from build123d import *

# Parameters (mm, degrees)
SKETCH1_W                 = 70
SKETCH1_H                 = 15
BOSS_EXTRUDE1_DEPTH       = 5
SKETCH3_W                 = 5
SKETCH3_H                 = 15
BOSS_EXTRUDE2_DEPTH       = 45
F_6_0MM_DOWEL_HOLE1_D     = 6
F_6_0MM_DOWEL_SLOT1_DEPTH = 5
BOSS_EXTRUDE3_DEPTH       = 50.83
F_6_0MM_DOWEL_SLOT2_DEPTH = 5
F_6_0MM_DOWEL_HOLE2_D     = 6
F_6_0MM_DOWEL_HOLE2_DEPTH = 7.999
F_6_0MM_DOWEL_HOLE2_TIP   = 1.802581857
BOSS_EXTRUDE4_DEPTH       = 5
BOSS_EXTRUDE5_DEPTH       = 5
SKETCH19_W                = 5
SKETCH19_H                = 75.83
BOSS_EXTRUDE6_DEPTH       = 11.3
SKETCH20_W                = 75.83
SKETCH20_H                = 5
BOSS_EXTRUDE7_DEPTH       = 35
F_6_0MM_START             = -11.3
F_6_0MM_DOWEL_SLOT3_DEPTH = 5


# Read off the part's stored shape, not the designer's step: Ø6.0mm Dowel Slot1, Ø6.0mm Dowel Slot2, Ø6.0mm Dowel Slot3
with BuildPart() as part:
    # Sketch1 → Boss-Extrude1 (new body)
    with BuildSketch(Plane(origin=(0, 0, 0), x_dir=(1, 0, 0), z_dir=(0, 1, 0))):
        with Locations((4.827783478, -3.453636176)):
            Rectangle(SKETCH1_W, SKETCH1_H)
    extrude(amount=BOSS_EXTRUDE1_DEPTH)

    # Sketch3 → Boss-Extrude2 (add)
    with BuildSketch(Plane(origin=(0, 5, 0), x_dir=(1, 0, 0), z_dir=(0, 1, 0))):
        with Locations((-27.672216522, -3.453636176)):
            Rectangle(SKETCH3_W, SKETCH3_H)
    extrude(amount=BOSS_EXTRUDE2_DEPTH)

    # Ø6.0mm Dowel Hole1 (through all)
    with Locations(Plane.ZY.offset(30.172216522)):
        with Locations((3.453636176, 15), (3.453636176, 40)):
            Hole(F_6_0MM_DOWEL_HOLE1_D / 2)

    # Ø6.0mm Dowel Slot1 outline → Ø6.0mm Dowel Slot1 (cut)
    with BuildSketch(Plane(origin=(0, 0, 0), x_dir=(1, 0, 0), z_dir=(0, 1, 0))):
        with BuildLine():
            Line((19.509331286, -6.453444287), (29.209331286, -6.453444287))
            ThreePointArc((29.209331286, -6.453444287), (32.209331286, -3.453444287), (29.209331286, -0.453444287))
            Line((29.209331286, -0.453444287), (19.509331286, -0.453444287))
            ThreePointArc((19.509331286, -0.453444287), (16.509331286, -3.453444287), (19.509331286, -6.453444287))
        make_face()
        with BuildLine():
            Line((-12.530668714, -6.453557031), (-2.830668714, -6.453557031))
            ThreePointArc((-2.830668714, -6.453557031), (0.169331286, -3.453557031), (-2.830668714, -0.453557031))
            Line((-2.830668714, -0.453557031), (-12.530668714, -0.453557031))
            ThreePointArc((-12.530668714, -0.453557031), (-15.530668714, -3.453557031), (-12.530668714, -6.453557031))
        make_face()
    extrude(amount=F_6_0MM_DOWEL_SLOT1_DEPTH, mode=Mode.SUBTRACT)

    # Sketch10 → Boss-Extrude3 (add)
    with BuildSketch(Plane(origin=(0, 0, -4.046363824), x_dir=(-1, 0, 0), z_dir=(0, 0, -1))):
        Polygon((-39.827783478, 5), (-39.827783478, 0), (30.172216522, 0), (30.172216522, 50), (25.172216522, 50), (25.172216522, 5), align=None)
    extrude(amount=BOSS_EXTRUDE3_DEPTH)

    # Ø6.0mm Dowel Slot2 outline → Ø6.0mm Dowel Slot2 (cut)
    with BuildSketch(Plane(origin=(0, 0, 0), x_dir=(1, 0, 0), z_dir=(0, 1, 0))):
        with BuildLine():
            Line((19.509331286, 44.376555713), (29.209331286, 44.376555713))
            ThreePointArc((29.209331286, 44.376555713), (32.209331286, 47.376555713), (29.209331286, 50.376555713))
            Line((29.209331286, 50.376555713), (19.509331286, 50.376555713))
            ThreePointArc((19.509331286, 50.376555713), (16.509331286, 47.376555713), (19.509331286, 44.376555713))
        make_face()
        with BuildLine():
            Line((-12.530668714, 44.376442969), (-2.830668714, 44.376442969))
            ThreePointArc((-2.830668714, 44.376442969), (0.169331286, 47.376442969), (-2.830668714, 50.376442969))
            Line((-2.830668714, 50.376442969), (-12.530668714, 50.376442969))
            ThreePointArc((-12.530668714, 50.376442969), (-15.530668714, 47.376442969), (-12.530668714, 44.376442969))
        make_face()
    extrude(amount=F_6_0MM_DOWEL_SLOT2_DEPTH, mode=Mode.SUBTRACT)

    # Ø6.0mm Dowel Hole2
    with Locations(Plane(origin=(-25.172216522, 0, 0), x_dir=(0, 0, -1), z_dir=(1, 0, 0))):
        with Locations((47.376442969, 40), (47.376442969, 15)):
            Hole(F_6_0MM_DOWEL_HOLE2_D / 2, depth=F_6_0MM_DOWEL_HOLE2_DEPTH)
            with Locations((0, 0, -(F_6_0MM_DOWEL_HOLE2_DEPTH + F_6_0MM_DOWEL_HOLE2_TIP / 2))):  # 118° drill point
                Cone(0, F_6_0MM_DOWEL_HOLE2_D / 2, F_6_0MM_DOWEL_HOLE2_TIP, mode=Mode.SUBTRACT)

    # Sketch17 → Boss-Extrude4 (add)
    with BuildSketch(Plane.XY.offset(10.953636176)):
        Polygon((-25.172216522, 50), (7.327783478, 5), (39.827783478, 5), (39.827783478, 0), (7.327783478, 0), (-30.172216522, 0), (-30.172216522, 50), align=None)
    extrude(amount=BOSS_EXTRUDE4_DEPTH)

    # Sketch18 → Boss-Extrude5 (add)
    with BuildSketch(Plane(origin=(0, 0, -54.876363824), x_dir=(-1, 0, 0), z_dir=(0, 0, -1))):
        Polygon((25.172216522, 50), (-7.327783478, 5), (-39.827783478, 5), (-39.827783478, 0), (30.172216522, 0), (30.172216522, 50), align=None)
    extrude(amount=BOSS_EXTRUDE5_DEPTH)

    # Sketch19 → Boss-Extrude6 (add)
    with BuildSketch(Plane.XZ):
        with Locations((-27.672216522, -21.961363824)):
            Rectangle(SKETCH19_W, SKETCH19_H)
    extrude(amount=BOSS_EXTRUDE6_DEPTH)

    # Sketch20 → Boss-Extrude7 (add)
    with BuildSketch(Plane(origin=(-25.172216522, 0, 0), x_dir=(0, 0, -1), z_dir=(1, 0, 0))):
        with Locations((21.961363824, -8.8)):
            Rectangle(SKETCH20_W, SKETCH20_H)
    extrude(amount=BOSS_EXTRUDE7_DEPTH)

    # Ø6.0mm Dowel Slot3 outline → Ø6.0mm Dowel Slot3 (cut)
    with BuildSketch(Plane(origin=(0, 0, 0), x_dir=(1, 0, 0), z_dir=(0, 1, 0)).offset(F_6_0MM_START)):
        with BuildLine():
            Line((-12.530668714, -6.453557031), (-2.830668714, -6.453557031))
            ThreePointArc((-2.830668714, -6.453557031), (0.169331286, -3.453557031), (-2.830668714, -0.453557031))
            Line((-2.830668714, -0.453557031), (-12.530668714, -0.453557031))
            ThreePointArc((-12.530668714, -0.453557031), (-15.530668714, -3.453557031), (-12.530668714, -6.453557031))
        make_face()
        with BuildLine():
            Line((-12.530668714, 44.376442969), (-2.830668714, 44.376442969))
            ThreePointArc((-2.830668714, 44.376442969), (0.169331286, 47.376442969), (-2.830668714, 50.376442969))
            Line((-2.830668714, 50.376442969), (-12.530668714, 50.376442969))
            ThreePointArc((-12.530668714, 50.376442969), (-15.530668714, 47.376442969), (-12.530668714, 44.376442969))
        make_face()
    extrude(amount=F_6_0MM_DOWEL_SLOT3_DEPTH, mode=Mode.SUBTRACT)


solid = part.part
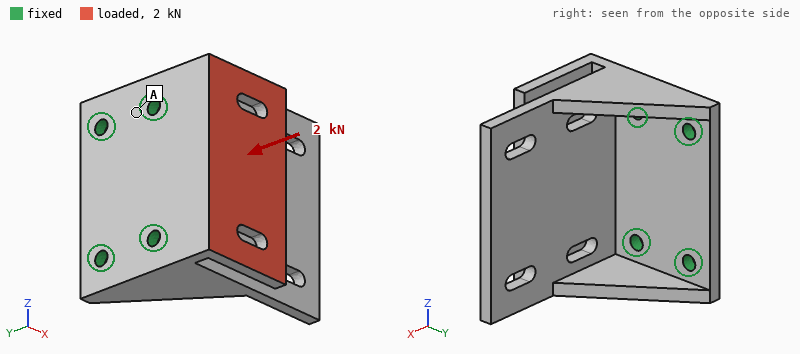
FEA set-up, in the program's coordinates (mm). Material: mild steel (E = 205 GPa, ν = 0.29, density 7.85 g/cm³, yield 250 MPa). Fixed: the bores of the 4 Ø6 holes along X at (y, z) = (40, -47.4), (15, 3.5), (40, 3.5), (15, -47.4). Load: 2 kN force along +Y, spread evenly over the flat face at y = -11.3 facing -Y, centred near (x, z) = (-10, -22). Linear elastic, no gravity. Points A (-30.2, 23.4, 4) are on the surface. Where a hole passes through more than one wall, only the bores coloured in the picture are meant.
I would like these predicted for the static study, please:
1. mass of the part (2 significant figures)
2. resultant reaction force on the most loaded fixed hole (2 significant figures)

510 g
840 N
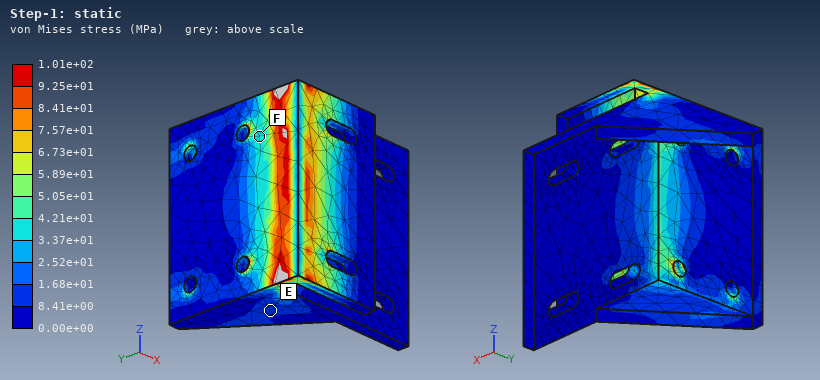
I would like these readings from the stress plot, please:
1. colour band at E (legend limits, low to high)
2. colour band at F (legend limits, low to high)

8.41e+00 to 1.68e+01 MPa
3.37e+01 to 4.21e+01 MPa
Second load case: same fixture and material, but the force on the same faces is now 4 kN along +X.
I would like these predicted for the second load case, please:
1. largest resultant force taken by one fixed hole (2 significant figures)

3.5 kN
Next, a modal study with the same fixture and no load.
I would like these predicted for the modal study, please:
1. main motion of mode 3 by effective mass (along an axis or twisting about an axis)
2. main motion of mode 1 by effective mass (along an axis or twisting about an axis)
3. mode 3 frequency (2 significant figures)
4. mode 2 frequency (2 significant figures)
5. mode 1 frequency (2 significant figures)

along Z
along Y
2900 Hz
2000 Hz
1500 Hz
